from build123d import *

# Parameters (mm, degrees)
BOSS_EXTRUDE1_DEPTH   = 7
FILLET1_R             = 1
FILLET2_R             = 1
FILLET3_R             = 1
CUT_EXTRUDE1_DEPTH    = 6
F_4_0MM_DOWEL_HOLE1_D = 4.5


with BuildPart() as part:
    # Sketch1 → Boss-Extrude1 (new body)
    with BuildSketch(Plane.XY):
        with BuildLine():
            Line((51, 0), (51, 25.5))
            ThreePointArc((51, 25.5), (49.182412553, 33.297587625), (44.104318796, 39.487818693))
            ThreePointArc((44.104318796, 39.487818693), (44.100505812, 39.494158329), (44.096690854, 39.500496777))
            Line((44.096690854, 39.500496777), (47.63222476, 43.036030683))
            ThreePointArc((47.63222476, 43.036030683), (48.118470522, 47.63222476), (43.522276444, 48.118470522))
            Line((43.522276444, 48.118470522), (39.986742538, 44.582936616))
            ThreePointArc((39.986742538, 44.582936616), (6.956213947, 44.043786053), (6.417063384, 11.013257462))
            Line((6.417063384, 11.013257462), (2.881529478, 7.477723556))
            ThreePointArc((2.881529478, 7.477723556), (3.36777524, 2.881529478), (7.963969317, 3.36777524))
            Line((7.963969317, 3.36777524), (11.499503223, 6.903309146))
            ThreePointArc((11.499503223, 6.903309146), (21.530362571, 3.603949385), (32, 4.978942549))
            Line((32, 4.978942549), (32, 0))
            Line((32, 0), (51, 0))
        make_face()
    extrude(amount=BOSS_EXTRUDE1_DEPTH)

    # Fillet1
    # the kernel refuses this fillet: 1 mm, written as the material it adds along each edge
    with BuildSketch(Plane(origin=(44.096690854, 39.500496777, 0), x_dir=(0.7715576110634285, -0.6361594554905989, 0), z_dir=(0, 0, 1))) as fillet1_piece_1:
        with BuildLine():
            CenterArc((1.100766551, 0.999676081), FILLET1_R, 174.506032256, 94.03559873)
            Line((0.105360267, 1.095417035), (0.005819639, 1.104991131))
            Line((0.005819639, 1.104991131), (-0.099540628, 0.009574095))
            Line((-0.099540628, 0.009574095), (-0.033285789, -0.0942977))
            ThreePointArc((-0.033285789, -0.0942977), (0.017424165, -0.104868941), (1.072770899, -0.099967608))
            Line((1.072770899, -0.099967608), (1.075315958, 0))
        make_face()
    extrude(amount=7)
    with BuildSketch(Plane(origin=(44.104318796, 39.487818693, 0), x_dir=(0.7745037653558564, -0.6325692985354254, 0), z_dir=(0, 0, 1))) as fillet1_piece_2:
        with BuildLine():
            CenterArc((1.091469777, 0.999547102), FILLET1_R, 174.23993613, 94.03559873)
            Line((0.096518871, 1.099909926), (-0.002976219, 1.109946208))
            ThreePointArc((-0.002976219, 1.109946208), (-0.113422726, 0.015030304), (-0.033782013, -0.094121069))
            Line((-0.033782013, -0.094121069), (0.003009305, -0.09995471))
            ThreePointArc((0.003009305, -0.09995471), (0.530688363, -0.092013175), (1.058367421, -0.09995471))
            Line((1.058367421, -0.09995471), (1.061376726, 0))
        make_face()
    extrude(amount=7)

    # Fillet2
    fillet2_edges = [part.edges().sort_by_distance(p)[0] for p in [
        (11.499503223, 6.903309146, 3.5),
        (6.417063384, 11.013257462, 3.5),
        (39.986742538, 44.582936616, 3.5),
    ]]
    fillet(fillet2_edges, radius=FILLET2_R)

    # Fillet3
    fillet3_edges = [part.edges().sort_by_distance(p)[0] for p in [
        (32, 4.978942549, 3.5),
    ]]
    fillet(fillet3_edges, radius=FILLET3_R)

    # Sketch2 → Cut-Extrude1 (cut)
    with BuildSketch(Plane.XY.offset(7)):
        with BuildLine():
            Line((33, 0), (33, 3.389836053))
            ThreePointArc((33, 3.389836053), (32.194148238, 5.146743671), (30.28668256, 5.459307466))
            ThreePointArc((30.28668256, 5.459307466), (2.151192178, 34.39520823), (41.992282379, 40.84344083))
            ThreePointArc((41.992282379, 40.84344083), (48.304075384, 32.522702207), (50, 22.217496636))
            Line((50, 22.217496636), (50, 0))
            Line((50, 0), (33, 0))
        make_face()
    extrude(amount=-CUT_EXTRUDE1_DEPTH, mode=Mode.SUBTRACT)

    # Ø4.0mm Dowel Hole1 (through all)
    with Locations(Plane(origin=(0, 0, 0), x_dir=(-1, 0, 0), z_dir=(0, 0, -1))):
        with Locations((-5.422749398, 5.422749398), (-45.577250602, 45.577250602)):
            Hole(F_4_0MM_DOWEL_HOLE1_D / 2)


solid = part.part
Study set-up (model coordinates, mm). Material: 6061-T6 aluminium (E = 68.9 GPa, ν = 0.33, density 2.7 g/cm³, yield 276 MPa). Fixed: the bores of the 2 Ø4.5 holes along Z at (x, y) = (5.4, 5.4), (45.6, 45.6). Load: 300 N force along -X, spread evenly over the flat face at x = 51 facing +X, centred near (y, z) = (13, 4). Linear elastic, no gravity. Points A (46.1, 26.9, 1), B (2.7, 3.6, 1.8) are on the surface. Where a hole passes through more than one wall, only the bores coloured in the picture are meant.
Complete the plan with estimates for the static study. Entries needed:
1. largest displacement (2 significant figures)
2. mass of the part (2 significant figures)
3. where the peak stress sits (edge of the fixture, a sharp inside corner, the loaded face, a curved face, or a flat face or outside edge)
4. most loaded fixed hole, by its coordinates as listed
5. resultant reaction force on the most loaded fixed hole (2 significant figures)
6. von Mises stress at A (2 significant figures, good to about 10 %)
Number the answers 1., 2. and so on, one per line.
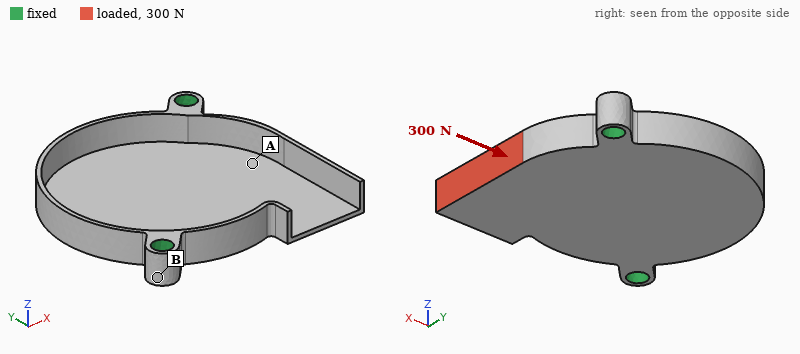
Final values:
1. 0.38 mm
2. 9.3 g
3. a curved face
4. (5.4, 5.4)
5. 220 N
6. 42 MPa
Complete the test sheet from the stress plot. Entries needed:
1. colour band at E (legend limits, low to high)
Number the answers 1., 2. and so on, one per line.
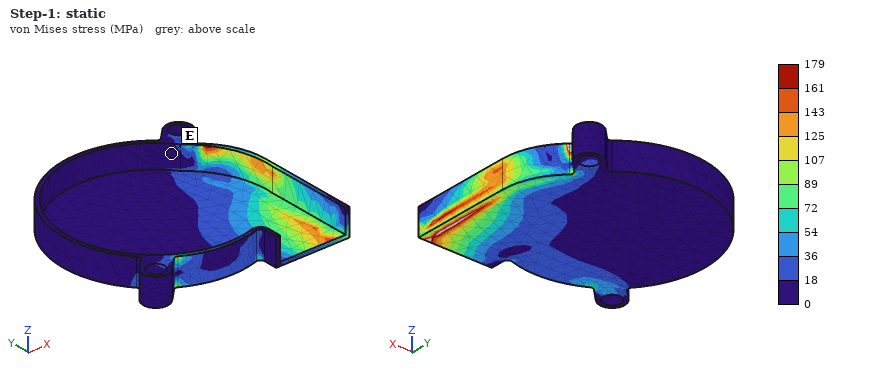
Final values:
1. 0 to 18 MPa
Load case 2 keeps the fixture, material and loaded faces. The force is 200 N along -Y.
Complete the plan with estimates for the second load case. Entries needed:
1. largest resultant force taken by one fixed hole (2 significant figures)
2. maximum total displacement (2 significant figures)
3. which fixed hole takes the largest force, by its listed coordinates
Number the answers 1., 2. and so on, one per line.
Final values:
1. 200 N
2. 0.17 mm
3. (45.6, 45.6)
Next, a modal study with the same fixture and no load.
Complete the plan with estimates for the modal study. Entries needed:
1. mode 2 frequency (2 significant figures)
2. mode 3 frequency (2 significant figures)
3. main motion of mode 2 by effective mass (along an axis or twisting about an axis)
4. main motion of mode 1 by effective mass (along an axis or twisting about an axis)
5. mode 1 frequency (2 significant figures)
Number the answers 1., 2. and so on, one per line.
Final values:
1. 3000 Hz
2. 4100 Hz
3. along Z
4. along Z
5. 2100 Hz
